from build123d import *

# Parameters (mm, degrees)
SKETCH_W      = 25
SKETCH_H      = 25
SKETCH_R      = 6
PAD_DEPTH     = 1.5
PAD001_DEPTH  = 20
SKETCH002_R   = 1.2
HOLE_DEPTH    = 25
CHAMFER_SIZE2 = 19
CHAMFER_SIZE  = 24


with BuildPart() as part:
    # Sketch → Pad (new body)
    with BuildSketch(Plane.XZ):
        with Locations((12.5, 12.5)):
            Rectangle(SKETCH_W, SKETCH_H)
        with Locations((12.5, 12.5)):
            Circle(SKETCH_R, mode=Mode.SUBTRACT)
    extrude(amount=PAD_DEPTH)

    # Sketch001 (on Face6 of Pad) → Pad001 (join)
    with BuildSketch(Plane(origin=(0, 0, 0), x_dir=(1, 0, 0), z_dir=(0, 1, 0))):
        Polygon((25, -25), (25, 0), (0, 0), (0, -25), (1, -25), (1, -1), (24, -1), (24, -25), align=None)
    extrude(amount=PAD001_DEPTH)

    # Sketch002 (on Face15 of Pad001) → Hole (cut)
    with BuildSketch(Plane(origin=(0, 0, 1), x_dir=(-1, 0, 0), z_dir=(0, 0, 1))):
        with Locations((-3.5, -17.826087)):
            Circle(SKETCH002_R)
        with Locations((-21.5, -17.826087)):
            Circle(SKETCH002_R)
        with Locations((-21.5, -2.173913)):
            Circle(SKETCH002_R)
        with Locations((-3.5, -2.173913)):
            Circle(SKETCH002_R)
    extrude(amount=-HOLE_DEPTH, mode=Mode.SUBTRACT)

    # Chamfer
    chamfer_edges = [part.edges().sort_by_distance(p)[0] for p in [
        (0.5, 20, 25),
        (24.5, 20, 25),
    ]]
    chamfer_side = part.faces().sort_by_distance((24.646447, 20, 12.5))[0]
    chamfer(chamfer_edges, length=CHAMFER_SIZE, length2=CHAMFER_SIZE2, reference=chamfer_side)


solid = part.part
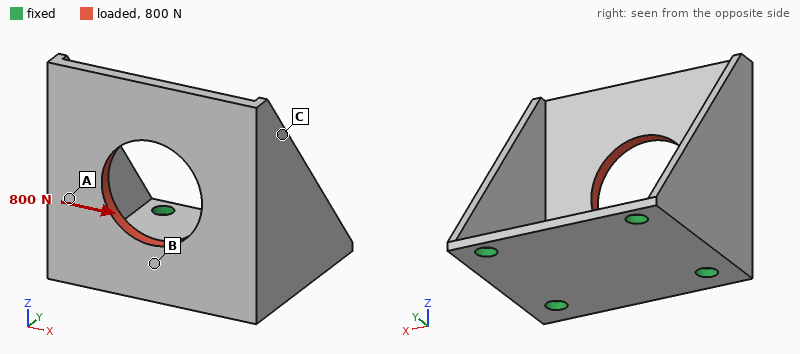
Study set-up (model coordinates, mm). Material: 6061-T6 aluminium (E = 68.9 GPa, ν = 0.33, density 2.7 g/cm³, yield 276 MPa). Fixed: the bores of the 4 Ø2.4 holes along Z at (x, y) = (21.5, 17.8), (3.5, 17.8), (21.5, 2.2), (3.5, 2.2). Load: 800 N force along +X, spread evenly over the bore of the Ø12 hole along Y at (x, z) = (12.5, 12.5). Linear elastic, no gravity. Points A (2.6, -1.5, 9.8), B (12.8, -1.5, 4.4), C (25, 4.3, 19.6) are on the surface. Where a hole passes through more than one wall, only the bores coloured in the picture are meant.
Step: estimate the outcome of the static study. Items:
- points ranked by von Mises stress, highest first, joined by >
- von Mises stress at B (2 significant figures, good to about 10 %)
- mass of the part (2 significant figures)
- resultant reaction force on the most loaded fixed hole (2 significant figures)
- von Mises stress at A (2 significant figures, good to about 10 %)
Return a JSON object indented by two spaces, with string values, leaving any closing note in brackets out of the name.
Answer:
{
  "points ranked by von Mises stress, highest first, joined by >": "B > A > C",
  "von Mises stress at B": "68 MPa",
  "mass of the part": "4.7 g",
  "resultant reaction force on the most loaded fixed hole": "660 N",
  "von Mises stress at A": "38 MPa"
}
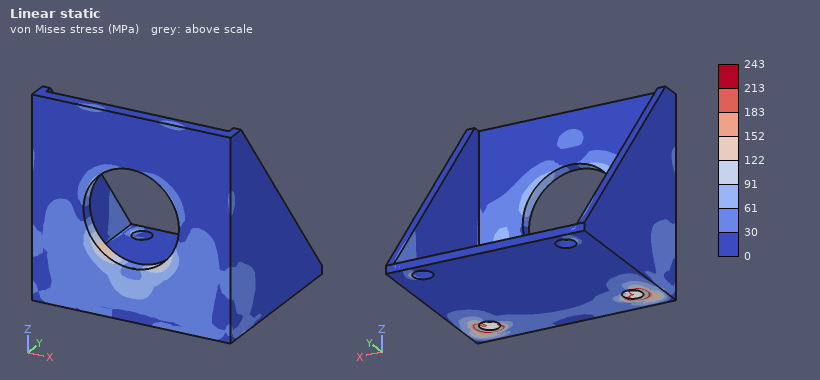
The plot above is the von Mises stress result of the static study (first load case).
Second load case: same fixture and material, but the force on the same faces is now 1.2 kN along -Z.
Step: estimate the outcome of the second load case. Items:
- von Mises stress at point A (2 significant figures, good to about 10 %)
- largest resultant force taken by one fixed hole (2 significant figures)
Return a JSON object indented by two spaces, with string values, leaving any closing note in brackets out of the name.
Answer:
{
  "von Mises stress at point A": "36 MPa",
  "largest resultant force taken by one fixed hole": "670 N"
}
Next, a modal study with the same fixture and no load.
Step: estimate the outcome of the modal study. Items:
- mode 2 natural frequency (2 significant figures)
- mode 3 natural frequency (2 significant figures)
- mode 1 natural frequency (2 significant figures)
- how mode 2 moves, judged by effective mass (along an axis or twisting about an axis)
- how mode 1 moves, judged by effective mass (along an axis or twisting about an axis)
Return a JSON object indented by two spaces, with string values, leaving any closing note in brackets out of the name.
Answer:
{
  "mode 2 natural frequency": "8500 Hz",
  "mode 3 natural frequency": "11 kHz",
  "mode 1 natural frequency": "6000 Hz",
  "how mode 2 moves, judged by effective mass": "along X",
  "how mode 1 moves, judged by effective mass": "along Y"
}
